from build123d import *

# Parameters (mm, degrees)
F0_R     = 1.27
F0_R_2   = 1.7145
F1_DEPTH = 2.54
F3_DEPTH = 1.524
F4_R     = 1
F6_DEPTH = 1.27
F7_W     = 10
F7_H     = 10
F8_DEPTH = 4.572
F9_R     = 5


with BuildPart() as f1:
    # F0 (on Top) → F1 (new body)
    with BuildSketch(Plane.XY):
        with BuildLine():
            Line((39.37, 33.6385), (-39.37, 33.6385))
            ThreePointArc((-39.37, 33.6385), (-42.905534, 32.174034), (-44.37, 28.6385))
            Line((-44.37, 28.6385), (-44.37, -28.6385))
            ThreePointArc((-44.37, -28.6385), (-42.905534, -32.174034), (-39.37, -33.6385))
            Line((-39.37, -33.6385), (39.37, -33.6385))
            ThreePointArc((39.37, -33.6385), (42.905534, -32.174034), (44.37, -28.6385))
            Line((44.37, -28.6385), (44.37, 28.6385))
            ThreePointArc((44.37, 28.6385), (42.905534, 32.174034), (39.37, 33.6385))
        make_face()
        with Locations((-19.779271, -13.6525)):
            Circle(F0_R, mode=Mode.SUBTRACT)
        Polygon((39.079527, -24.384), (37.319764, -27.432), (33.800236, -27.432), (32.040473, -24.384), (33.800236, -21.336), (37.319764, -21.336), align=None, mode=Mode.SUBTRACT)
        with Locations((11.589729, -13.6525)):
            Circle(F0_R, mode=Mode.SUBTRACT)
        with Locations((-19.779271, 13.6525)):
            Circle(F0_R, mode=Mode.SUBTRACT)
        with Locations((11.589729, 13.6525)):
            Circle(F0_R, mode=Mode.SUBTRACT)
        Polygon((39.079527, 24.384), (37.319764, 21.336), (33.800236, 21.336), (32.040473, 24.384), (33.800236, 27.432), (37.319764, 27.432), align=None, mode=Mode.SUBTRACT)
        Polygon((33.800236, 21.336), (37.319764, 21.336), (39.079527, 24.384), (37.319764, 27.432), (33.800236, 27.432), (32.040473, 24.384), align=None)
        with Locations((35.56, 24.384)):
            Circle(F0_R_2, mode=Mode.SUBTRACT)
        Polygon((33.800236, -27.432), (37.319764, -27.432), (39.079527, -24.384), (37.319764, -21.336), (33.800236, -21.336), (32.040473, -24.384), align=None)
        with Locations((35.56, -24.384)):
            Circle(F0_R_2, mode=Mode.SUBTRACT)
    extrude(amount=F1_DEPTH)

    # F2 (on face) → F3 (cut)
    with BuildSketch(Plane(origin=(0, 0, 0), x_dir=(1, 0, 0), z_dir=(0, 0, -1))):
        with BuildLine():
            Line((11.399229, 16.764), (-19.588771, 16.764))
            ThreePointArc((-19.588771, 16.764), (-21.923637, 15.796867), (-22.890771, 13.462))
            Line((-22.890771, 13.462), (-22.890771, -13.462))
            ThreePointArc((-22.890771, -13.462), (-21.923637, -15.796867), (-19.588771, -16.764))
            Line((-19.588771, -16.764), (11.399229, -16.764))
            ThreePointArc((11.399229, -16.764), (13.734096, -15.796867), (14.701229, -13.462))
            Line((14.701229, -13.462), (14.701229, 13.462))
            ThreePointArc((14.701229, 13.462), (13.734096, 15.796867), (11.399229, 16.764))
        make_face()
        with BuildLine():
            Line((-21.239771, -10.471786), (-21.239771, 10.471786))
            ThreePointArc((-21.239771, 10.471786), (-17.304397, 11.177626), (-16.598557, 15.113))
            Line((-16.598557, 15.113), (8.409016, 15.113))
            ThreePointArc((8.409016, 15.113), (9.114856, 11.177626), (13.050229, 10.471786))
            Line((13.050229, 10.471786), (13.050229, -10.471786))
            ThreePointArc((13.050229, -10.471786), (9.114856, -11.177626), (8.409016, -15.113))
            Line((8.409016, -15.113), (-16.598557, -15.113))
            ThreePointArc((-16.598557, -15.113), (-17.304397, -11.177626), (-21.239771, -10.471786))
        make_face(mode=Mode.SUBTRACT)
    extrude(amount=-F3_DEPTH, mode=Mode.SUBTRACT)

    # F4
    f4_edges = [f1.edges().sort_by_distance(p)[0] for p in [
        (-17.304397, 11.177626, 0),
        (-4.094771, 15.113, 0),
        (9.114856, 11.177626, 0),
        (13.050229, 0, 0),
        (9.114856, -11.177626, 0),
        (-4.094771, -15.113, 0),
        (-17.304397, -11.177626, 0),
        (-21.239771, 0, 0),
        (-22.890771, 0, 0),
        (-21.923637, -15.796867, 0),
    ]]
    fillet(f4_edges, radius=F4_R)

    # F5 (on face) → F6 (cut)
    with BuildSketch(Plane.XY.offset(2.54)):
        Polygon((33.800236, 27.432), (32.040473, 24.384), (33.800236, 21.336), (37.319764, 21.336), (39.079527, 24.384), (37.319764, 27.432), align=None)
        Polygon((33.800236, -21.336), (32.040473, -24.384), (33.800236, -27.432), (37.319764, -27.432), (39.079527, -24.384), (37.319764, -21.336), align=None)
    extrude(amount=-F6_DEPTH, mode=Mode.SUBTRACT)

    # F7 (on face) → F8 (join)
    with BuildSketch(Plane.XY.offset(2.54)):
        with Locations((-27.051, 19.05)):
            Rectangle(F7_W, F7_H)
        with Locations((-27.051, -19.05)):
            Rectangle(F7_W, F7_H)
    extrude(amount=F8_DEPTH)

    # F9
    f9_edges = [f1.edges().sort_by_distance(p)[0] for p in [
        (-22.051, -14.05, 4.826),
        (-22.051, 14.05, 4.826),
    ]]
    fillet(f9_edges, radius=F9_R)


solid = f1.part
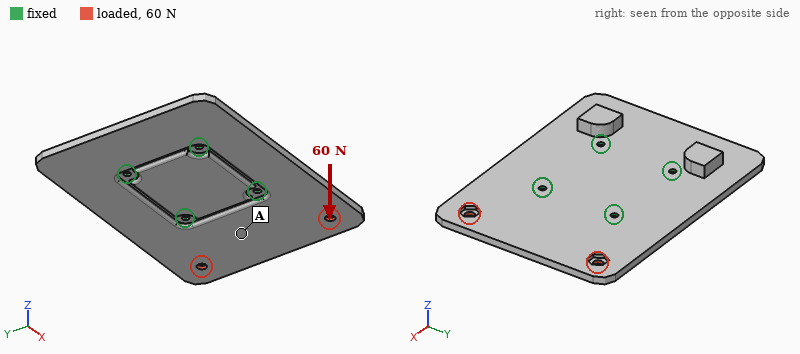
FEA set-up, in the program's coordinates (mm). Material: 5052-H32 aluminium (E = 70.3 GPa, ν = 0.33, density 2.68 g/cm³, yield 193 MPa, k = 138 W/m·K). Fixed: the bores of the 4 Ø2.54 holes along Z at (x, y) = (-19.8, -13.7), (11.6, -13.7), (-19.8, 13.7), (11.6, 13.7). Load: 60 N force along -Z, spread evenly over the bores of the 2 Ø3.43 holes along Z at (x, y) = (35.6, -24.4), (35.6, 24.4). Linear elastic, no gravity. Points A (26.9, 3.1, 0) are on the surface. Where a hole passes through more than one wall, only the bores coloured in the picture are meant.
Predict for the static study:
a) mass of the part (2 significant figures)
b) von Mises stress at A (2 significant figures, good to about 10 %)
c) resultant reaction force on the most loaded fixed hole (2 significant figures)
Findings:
41 g
6.5 MPa
130 N
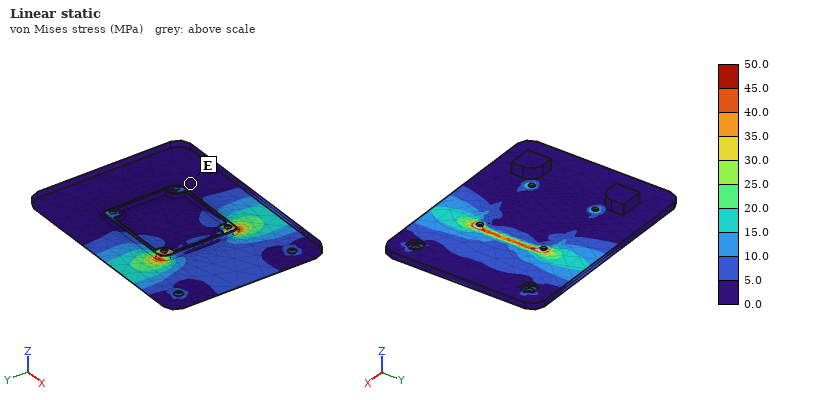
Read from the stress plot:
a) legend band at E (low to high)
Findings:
0.0 to 5.0 MPa
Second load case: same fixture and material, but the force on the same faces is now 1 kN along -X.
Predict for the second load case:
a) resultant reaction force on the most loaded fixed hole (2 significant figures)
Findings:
280 N
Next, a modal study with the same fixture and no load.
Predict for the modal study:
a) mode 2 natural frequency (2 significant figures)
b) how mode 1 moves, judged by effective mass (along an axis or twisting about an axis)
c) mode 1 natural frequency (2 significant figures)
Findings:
2000 Hz
along Z
1300 Hz
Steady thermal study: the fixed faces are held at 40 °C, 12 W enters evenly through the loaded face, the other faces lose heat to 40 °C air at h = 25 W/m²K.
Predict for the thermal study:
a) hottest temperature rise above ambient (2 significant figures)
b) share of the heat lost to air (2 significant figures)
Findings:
25 K
18 %
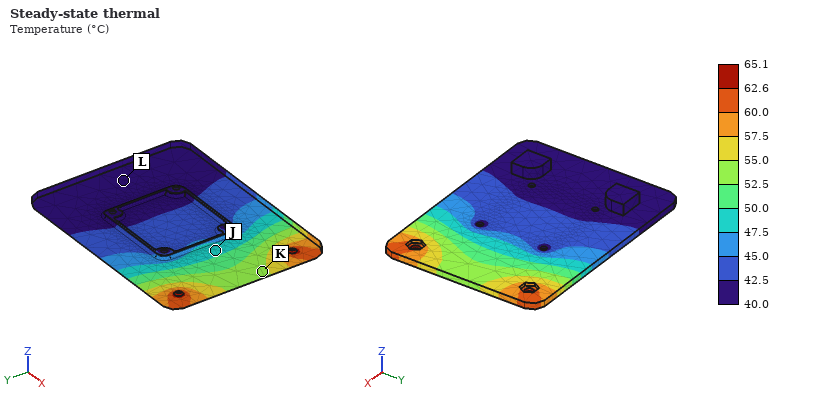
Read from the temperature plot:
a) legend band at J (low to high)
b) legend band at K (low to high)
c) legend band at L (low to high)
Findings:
47.5 to 50.0 °C
52.5 to 55.0 °C
40.0 to 42.5 °C
